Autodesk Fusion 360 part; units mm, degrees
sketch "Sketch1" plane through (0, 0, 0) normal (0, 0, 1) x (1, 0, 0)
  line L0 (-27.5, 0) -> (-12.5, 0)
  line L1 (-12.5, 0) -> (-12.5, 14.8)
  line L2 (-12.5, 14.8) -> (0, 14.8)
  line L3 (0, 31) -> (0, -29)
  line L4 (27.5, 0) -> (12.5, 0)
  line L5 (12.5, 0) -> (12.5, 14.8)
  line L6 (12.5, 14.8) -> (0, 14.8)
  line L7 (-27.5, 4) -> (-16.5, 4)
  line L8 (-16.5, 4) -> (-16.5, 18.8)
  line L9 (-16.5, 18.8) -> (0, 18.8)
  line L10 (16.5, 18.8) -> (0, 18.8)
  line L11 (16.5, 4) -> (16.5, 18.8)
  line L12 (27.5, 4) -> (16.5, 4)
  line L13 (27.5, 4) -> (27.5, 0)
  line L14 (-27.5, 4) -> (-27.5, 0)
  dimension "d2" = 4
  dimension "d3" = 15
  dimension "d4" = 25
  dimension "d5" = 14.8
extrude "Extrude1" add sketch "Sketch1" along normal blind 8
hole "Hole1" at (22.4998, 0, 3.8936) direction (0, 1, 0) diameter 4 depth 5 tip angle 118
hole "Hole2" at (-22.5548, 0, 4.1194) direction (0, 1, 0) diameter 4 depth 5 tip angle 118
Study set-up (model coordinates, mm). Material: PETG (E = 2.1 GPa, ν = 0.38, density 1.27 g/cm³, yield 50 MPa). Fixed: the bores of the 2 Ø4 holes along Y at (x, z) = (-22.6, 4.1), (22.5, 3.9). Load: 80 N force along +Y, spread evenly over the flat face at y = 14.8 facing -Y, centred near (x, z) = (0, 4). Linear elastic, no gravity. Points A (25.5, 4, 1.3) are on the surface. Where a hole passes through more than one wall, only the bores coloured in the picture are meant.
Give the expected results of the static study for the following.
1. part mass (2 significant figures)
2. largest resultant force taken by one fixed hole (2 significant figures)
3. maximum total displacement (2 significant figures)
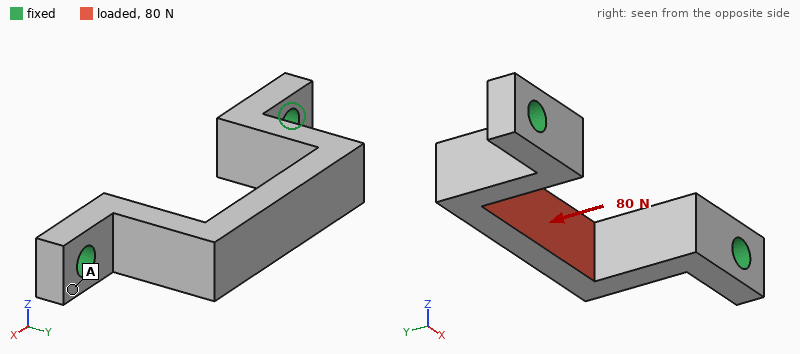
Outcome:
3.3 g
46 N
0.13 mm
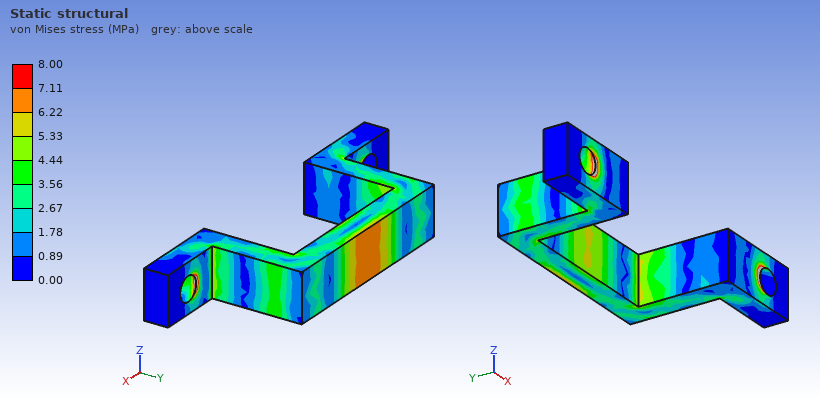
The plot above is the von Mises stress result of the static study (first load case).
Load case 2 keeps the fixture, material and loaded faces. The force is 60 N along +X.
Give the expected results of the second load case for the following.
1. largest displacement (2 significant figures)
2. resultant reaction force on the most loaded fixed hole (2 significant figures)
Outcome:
0.23 mm
32 N
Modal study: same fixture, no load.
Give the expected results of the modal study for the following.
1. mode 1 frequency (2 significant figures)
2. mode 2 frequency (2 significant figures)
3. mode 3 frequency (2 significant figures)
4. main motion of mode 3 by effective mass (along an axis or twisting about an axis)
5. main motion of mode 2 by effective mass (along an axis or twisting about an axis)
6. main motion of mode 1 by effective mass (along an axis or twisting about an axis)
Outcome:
1400 Hz
2100 Hz
2600 Hz
twisting about Y
along X
along Z
